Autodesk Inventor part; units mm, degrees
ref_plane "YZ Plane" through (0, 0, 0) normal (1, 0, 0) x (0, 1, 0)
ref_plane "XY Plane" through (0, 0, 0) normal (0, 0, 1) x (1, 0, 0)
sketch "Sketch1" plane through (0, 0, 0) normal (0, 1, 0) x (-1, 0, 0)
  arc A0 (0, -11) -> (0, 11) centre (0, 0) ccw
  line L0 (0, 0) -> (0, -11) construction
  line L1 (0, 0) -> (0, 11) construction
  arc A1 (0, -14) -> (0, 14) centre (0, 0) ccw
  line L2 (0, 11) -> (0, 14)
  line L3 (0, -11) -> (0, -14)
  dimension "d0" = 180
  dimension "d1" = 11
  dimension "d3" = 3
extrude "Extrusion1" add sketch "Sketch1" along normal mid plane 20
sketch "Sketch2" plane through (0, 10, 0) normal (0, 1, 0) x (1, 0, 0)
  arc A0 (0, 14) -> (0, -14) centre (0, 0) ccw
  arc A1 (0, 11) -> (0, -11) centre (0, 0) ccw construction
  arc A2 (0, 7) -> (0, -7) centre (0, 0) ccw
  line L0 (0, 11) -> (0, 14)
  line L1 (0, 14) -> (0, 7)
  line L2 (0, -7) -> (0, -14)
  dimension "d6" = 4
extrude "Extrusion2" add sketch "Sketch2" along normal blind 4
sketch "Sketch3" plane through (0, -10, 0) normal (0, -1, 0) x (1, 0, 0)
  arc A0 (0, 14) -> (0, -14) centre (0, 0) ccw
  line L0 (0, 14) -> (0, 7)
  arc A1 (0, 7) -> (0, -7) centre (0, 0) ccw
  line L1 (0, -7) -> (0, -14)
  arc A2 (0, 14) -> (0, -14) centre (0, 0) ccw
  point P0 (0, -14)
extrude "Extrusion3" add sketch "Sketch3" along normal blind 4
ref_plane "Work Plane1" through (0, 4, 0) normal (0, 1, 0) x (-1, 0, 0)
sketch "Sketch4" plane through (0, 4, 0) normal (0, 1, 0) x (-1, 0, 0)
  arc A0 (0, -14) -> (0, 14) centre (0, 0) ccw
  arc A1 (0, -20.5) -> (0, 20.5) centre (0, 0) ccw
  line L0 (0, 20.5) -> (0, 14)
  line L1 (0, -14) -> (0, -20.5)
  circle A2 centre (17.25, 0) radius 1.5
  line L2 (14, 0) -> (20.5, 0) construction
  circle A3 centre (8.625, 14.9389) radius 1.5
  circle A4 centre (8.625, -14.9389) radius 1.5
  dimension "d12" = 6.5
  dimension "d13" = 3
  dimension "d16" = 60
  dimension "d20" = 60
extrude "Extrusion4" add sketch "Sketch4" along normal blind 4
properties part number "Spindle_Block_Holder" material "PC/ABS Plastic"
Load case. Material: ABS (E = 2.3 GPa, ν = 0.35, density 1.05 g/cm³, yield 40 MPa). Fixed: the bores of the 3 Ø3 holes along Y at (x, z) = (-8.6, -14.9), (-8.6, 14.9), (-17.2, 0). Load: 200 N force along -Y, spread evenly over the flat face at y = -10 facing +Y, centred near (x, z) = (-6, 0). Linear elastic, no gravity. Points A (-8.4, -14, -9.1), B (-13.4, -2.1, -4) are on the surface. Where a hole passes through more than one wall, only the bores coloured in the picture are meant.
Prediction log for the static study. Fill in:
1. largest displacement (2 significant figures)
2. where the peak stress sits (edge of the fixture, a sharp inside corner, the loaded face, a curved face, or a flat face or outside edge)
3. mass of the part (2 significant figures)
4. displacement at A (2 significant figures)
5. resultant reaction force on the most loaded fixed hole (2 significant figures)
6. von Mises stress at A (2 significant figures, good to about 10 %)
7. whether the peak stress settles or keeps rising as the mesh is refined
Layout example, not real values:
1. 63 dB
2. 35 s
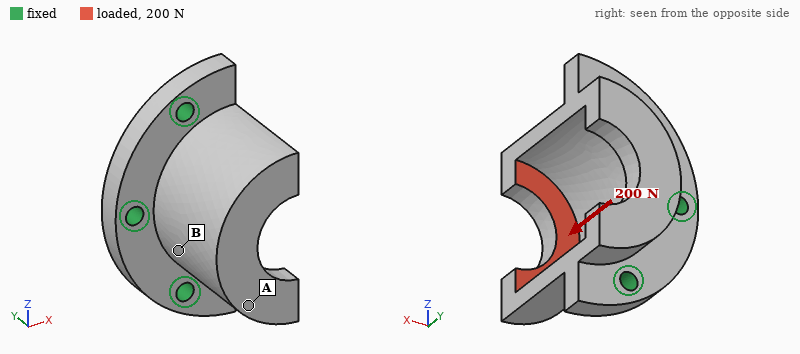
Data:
1. 0.16 mm
2. edge of the fixture
3. 5.8 g
4. 0.11 mm
5. 96 N
6. 3.1 MPa
7. keeps rising
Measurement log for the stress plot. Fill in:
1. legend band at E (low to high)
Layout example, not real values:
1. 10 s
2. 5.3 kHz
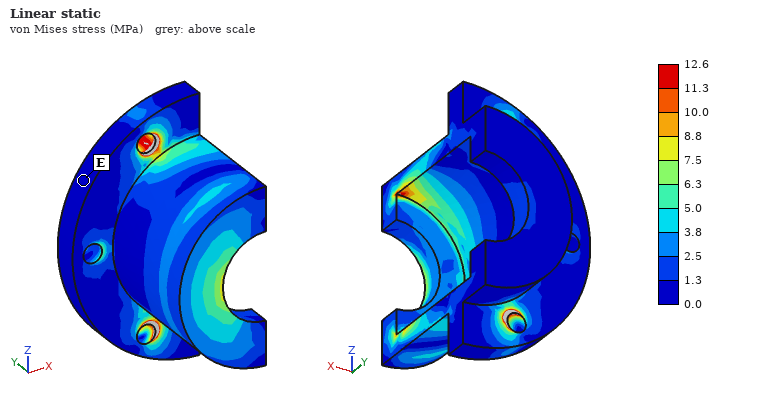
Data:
1. 0.0 to 1.3 MPa
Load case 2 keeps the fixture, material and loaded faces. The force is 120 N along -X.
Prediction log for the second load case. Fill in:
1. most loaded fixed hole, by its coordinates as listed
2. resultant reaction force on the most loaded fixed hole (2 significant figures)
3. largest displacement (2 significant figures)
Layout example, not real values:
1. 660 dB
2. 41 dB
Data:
1. (-17.2, 0)
2. 150 N
3. 0.24 mm
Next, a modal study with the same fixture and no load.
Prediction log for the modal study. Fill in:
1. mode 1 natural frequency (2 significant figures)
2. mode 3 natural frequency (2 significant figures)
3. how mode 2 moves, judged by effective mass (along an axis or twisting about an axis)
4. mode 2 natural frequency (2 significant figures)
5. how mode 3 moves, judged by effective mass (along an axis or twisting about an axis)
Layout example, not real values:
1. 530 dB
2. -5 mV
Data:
1. 2700 Hz
2. 5300 Hz
3. along X
4. 2800 Hz
5. along Z
